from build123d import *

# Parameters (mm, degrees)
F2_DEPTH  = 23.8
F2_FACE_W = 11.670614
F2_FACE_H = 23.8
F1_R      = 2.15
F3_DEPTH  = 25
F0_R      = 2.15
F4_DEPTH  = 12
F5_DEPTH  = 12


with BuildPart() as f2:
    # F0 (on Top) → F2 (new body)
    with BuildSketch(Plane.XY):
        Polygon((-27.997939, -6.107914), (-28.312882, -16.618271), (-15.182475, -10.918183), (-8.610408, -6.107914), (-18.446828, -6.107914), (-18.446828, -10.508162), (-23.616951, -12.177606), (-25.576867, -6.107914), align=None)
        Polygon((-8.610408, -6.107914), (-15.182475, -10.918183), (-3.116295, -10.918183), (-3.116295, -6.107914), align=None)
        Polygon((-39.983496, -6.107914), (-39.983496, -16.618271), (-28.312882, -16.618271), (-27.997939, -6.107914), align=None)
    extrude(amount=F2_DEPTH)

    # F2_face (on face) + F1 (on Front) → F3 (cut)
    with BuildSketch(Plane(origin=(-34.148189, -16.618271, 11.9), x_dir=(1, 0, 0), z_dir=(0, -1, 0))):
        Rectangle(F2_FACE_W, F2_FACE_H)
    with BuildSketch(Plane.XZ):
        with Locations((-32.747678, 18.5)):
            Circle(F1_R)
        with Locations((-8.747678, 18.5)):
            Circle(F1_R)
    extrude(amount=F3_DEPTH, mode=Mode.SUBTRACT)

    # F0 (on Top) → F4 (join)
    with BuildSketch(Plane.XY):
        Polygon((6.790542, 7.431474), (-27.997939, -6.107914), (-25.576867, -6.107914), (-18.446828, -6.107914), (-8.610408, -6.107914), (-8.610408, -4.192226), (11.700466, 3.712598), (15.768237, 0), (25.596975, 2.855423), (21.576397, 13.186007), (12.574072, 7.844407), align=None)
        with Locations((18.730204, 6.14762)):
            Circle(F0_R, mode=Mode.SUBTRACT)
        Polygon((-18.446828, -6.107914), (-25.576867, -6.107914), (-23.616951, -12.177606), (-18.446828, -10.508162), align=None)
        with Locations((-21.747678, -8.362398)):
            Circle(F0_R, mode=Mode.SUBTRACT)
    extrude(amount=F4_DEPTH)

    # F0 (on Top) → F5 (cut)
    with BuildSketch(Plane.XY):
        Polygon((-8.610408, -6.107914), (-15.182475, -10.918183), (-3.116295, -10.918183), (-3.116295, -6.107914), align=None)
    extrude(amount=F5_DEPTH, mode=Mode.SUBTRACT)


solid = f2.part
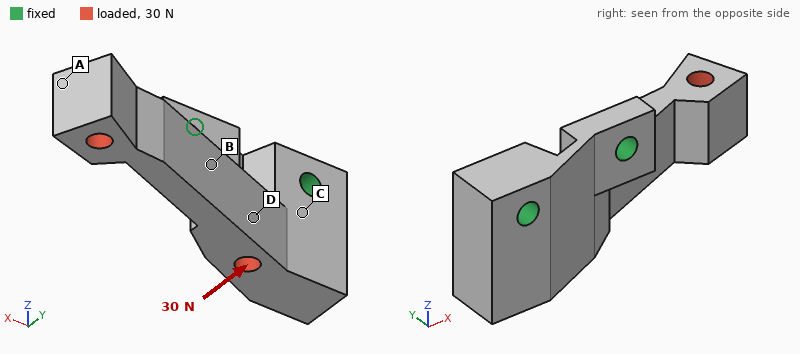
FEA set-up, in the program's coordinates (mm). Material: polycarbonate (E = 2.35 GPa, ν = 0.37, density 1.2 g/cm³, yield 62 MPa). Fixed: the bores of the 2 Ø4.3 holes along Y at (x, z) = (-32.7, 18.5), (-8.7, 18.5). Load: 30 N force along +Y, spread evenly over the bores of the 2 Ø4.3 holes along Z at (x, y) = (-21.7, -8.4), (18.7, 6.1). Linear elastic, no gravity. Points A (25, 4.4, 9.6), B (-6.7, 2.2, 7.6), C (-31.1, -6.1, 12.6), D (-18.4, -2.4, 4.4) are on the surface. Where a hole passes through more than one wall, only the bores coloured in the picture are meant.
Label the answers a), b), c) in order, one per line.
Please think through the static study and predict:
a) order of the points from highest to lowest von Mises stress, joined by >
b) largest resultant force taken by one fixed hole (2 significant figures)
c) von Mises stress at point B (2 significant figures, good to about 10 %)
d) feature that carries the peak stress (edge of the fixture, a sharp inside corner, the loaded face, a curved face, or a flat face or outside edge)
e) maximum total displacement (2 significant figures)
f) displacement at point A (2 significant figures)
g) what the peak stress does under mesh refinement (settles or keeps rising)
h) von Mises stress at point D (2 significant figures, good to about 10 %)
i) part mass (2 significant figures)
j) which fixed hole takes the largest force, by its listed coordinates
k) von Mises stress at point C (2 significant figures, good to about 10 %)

a) B > D > C > A
b) 32 N
c) 6.5 MPa
d) a sharp inside corner
e) 0.82 mm
f) 0.78 mm
g) keeps rising
h) 2.6 MPa
i) 11 g
j) (-8.7, 18.5)
k) 1.3 MPa
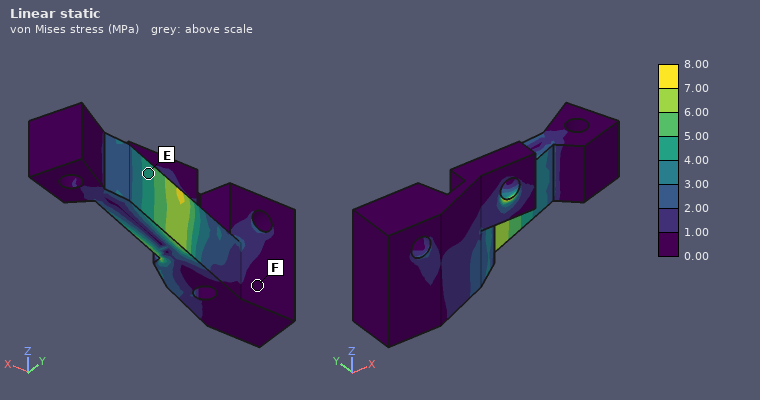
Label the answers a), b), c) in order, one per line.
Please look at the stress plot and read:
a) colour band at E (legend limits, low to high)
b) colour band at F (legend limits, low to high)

a) 4.00 to 5.00 MPa
b) 0.00 to 1.00 MPa
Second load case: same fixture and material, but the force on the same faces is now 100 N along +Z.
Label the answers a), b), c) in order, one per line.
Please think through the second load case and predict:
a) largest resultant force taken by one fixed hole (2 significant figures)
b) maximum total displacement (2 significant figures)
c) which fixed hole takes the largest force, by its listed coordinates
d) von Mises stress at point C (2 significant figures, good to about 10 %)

a) 130 N
b) 0.86 mm
c) (-8.7, 18.5)
d) 1.7 MPa
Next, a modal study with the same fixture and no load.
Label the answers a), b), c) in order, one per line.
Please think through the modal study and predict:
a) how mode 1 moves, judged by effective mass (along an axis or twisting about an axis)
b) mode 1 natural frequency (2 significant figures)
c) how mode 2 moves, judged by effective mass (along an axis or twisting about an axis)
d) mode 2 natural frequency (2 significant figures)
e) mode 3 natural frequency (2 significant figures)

a) along Y
b) 590 Hz
c) along Z
d) 1100 Hz
e) 2400 Hz
